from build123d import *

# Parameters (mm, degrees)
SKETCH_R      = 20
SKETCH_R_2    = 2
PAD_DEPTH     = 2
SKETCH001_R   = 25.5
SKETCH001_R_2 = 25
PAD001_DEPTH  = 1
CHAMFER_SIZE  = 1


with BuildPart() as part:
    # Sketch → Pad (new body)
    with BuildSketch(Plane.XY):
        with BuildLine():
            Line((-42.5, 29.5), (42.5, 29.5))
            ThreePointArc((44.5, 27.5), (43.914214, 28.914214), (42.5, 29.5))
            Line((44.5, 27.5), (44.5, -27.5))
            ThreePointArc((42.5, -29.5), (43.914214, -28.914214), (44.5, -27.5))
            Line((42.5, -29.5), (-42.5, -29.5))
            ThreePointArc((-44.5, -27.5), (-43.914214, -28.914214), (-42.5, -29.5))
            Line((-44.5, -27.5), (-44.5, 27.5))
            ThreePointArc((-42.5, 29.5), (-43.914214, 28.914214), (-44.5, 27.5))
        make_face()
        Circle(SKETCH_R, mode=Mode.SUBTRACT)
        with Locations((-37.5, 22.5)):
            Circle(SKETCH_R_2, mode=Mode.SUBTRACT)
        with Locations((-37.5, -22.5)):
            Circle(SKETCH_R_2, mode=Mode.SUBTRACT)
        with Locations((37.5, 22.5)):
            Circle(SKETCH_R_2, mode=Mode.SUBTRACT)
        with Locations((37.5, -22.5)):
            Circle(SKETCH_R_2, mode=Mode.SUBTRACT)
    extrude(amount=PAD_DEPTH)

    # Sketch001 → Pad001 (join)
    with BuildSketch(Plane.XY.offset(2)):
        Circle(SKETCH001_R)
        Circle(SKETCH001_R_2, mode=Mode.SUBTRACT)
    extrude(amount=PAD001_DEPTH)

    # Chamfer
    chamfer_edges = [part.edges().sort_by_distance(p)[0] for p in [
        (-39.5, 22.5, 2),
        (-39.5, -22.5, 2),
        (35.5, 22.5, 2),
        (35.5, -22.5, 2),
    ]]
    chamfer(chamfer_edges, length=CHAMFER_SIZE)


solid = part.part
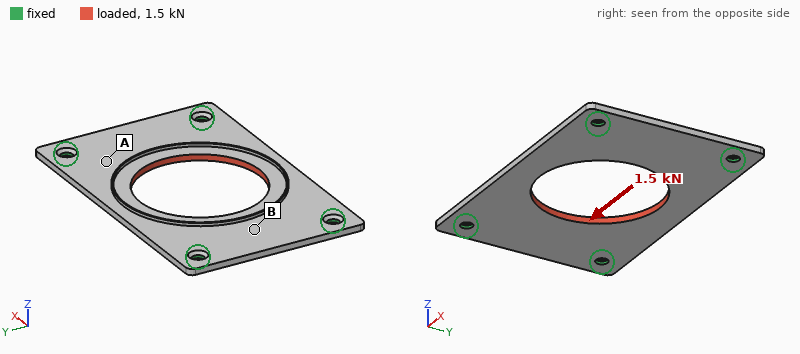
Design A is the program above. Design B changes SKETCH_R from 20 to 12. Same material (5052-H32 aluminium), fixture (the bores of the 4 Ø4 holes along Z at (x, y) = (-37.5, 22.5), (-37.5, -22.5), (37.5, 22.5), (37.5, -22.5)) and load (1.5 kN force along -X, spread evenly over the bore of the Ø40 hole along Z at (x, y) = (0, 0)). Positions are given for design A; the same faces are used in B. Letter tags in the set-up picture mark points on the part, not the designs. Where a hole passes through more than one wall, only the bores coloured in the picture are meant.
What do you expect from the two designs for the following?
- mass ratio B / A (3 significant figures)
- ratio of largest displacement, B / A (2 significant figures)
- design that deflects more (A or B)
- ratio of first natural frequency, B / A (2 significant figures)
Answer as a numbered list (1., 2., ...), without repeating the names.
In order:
1. 1.20
2. 0.92
3. A
4. 0.84
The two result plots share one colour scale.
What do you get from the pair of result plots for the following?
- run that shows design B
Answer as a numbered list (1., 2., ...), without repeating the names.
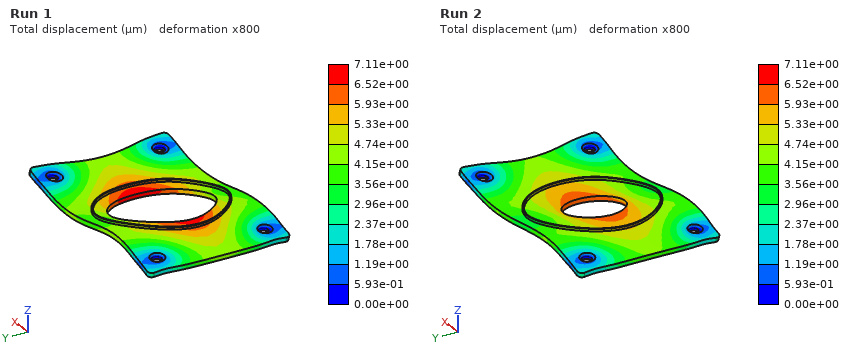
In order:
1. Run 2
